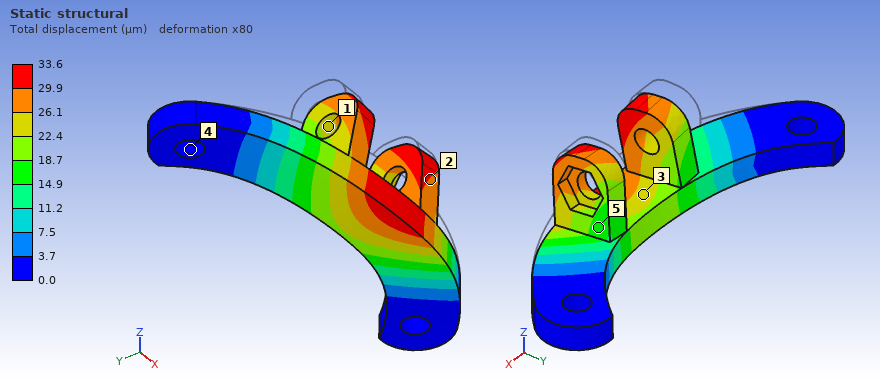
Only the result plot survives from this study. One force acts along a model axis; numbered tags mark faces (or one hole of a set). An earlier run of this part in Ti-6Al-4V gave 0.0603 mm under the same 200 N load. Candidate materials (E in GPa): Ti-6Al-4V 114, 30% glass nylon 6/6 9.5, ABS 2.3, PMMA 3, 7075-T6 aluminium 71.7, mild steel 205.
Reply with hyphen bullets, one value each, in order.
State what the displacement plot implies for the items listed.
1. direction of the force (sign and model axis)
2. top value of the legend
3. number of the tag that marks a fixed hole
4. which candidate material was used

- -Z
- 33.6 µm
- 4
- mild steel
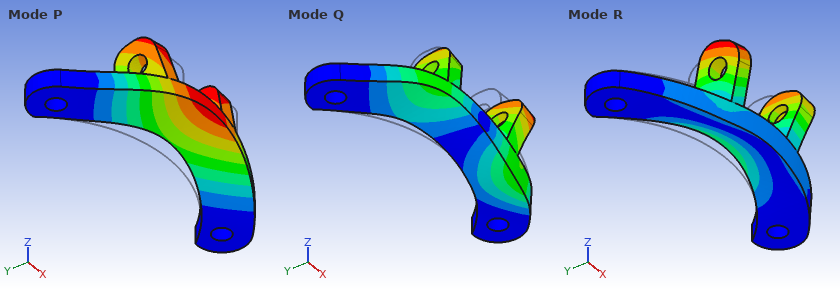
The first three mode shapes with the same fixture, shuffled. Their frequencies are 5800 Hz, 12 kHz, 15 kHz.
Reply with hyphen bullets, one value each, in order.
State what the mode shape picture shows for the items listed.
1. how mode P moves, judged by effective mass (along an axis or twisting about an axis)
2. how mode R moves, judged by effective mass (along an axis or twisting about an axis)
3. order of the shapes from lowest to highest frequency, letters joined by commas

- along Z
- along Y
- P, R, Q
